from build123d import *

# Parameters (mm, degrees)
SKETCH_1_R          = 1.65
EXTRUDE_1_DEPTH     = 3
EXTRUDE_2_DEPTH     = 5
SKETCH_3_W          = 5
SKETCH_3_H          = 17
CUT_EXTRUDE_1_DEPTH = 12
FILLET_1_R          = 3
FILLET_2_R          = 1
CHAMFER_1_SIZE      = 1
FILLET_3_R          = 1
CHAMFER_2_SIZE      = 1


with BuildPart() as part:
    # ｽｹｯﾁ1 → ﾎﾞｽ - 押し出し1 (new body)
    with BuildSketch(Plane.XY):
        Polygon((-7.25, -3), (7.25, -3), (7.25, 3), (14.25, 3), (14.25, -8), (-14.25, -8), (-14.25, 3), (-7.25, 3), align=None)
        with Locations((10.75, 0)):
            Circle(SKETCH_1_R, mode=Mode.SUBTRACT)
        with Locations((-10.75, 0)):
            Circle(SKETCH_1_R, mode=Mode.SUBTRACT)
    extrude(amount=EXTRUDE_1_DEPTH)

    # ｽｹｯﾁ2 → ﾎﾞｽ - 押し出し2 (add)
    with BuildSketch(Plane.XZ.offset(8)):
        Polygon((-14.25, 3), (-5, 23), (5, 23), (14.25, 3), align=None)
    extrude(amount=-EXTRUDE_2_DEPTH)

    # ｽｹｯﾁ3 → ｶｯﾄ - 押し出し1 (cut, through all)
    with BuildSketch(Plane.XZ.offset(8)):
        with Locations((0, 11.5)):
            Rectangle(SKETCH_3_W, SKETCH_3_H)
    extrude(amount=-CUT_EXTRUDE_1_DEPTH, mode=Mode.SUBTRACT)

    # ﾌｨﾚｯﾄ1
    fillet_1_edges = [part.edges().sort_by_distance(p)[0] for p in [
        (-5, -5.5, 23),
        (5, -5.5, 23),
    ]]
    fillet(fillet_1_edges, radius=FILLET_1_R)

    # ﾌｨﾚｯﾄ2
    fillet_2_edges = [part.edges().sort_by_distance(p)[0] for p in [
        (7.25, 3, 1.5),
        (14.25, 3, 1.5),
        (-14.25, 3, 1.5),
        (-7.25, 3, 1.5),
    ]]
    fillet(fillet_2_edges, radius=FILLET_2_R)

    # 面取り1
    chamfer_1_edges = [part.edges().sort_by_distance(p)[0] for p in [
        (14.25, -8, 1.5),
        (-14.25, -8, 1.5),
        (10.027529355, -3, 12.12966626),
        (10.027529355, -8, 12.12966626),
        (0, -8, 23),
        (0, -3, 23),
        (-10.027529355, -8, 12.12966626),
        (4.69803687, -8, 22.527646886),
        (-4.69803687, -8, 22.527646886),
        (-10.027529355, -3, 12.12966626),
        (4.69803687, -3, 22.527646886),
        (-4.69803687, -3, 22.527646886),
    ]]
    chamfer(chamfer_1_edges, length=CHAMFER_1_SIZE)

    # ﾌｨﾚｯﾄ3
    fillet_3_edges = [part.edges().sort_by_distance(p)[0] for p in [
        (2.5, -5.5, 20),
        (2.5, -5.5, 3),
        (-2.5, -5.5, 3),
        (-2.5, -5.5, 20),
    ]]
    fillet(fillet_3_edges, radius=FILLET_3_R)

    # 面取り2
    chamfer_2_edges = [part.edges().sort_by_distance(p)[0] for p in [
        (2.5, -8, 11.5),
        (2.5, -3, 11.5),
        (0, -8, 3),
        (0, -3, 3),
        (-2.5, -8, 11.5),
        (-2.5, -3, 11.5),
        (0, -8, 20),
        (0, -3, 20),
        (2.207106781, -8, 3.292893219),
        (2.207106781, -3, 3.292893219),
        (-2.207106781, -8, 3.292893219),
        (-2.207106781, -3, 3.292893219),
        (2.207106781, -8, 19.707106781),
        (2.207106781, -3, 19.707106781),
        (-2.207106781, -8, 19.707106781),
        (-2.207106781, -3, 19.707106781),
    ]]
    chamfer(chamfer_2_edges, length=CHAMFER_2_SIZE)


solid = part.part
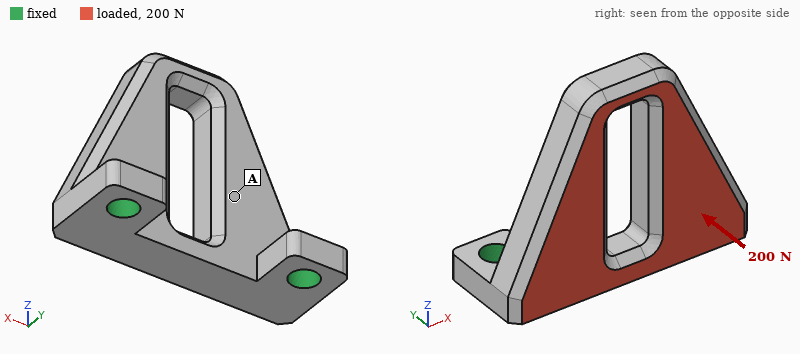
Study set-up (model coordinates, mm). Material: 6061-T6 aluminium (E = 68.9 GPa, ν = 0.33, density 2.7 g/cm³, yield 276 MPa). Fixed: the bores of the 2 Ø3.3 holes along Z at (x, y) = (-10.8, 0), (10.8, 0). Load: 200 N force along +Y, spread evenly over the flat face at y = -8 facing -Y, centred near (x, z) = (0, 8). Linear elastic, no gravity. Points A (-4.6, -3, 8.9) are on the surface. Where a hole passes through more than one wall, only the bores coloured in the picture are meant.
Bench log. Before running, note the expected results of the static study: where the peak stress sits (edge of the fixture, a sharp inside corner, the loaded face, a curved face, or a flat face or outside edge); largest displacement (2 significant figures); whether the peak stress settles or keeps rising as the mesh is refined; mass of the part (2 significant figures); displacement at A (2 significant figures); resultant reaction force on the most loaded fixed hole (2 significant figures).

edge of the fixture
55 µm
keeps rising
5.5 g
18 µm
110 N
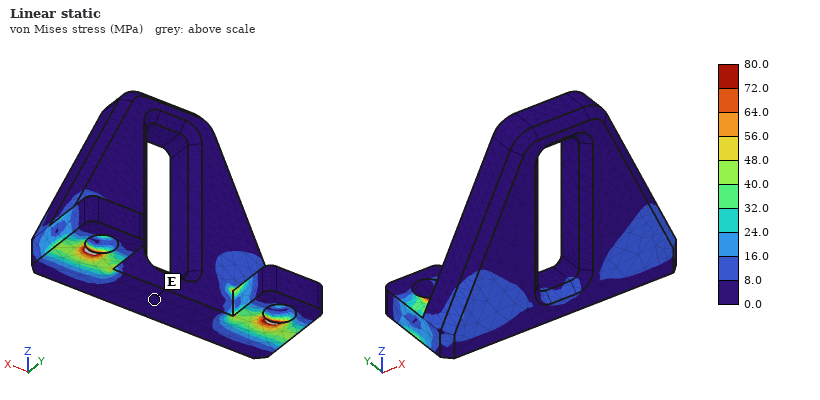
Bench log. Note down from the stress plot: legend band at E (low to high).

0.0 to 8.0 MPa
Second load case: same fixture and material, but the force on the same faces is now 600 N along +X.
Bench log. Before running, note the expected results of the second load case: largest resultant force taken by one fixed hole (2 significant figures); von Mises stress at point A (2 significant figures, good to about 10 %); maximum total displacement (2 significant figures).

360 N
6.7 MPa
16 µm
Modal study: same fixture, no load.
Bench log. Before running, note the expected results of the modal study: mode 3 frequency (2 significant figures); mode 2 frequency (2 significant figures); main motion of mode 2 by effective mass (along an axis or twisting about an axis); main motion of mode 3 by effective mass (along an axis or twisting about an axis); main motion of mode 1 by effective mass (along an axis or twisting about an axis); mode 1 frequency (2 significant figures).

20 kHz
14 kHz
along X
along X
along Y
5000 Hz
